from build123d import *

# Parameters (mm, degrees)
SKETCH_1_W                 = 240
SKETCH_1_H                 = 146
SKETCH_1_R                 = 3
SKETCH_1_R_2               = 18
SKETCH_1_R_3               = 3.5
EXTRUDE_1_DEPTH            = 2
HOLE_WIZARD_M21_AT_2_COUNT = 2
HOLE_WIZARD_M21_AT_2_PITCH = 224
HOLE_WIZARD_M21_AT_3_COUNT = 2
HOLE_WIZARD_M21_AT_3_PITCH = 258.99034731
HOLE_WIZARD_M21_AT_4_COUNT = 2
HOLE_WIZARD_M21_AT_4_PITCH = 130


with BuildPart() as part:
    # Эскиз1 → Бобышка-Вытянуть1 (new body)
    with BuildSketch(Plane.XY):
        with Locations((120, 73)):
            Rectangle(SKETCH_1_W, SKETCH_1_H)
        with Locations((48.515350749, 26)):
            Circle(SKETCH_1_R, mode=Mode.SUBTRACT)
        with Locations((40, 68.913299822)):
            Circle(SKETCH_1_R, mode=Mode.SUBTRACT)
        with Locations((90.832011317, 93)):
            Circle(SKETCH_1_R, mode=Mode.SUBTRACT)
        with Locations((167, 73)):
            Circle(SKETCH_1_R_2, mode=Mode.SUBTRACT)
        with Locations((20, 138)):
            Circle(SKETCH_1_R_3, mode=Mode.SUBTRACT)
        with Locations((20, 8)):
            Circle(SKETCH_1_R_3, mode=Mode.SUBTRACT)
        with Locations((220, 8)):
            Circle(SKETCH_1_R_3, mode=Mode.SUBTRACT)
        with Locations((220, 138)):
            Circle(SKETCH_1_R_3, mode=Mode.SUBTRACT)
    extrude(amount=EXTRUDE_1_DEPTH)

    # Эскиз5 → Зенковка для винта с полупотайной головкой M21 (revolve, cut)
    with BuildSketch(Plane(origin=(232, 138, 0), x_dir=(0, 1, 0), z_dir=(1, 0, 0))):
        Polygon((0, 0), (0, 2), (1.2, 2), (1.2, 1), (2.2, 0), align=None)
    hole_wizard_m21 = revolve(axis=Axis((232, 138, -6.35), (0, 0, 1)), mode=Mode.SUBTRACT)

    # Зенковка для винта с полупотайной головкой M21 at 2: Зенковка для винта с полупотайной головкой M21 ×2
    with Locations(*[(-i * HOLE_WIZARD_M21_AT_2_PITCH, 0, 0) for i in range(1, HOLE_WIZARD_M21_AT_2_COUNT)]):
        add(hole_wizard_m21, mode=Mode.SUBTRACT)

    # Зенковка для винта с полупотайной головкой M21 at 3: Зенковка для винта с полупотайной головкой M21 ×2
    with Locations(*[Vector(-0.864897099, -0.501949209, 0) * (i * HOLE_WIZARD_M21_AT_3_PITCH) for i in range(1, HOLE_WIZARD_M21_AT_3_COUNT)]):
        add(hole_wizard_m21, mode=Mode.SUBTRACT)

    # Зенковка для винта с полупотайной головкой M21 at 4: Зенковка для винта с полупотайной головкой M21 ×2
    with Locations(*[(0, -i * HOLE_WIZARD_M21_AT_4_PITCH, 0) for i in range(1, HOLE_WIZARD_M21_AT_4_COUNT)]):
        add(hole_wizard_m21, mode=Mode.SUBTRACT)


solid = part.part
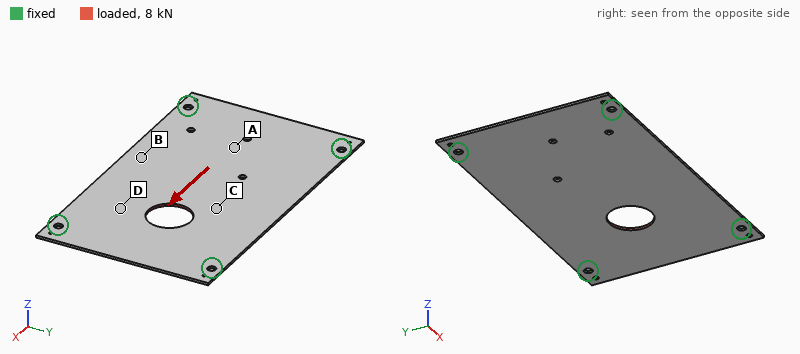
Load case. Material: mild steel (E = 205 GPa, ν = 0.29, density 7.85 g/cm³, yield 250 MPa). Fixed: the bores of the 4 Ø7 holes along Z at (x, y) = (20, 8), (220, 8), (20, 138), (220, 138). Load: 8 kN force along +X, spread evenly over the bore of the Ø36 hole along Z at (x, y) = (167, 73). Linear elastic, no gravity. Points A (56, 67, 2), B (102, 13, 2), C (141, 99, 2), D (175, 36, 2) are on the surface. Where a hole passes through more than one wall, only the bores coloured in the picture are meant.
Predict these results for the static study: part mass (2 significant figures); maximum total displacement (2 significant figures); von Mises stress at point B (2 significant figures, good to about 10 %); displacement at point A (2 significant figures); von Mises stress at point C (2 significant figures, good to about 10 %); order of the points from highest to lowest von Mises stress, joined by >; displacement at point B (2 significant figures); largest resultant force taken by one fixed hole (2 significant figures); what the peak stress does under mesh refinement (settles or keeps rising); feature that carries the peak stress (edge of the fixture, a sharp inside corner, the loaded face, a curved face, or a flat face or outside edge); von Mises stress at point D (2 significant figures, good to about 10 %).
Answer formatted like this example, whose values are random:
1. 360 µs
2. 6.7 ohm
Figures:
1. 530 g
2. 20 µm
3. 11 MPa
4. 7.5 µm
5. 29 MPa
6. C > D > B > A
7. 8.3 µm
8. 2.5 kN
9. keeps rising
10. edge of the fixture
11. 22 MPa
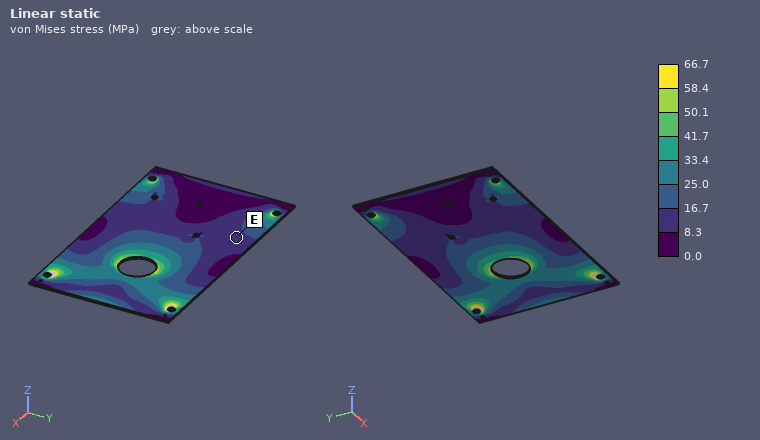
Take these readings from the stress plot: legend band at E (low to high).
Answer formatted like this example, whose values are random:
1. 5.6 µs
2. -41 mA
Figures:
1. 8.3 to 16.7 MPa
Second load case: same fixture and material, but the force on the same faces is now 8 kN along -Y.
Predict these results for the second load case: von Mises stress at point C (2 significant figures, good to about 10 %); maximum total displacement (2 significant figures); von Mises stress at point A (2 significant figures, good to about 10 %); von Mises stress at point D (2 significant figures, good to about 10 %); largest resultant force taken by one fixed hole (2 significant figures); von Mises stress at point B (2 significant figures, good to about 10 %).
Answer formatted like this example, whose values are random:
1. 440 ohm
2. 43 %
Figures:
1. 20 MPa
2. 25 µm
3. 15 MPa
4. 35 MPa
5. 3.1 kN
6. 10 MPa
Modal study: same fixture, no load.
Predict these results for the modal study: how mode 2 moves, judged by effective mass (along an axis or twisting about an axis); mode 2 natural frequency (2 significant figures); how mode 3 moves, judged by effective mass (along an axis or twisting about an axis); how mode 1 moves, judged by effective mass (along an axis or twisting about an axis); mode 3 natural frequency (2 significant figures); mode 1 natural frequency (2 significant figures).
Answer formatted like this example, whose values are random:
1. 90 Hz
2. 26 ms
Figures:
1. twisting about X
2. 350 Hz
3. twisting about Y
4. along Z
5. 540 Hz
6. 220 Hz
